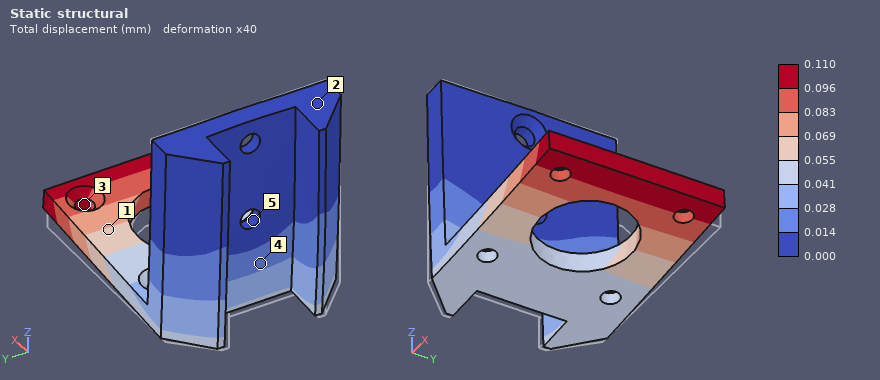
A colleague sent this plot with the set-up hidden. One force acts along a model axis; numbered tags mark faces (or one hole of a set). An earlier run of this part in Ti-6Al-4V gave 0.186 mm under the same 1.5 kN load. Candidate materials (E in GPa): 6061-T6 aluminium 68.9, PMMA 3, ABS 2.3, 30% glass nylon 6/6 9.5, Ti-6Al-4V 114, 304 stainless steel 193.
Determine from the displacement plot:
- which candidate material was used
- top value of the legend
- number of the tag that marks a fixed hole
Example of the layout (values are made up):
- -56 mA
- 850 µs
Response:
- 304 stainless steel
- 0.110 mm
- 5
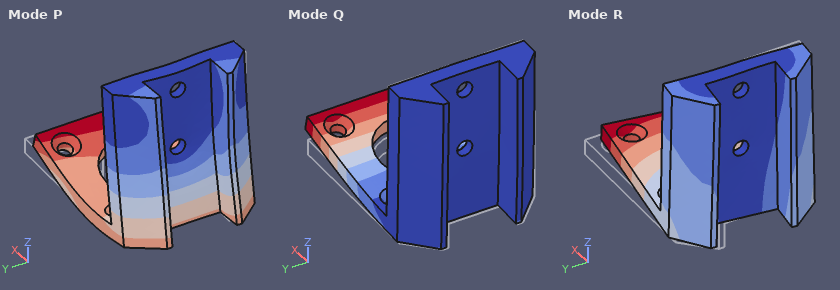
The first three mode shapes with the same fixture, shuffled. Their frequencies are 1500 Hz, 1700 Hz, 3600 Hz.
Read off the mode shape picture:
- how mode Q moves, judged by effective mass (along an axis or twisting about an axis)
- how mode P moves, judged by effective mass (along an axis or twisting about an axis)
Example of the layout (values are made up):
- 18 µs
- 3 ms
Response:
- along Z
- along X
